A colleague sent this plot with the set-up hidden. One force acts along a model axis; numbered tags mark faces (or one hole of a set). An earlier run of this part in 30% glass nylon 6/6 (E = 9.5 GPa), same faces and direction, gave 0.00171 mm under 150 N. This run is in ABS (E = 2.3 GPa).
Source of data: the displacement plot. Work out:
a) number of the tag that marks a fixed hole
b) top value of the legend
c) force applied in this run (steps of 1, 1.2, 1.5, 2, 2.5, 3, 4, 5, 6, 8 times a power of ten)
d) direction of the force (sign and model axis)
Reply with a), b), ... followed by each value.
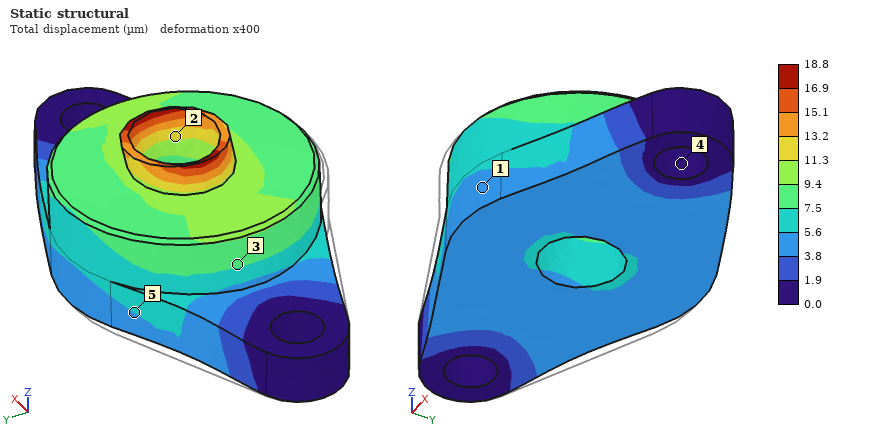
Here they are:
a) 4
b) 18.8 µm
c) 400 N
d) +X
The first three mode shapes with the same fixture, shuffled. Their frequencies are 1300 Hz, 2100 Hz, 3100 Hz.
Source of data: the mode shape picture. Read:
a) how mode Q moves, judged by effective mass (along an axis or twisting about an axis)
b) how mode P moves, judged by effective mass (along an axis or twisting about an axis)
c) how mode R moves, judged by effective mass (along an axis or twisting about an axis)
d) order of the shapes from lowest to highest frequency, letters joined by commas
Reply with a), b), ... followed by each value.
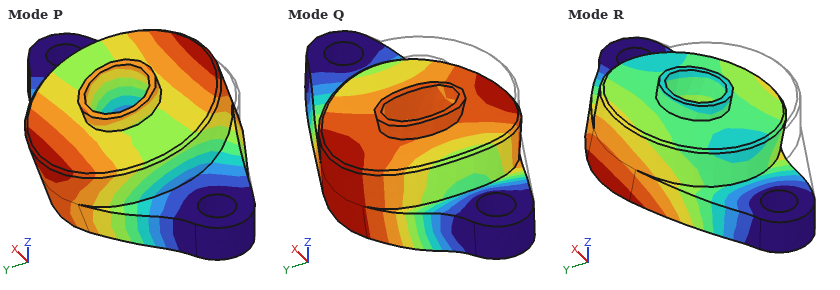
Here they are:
a) along Z
b) along Y
c) along Y
d) P, Q, R
